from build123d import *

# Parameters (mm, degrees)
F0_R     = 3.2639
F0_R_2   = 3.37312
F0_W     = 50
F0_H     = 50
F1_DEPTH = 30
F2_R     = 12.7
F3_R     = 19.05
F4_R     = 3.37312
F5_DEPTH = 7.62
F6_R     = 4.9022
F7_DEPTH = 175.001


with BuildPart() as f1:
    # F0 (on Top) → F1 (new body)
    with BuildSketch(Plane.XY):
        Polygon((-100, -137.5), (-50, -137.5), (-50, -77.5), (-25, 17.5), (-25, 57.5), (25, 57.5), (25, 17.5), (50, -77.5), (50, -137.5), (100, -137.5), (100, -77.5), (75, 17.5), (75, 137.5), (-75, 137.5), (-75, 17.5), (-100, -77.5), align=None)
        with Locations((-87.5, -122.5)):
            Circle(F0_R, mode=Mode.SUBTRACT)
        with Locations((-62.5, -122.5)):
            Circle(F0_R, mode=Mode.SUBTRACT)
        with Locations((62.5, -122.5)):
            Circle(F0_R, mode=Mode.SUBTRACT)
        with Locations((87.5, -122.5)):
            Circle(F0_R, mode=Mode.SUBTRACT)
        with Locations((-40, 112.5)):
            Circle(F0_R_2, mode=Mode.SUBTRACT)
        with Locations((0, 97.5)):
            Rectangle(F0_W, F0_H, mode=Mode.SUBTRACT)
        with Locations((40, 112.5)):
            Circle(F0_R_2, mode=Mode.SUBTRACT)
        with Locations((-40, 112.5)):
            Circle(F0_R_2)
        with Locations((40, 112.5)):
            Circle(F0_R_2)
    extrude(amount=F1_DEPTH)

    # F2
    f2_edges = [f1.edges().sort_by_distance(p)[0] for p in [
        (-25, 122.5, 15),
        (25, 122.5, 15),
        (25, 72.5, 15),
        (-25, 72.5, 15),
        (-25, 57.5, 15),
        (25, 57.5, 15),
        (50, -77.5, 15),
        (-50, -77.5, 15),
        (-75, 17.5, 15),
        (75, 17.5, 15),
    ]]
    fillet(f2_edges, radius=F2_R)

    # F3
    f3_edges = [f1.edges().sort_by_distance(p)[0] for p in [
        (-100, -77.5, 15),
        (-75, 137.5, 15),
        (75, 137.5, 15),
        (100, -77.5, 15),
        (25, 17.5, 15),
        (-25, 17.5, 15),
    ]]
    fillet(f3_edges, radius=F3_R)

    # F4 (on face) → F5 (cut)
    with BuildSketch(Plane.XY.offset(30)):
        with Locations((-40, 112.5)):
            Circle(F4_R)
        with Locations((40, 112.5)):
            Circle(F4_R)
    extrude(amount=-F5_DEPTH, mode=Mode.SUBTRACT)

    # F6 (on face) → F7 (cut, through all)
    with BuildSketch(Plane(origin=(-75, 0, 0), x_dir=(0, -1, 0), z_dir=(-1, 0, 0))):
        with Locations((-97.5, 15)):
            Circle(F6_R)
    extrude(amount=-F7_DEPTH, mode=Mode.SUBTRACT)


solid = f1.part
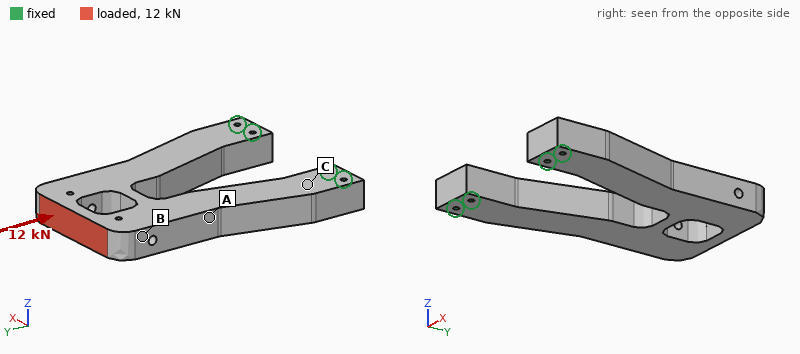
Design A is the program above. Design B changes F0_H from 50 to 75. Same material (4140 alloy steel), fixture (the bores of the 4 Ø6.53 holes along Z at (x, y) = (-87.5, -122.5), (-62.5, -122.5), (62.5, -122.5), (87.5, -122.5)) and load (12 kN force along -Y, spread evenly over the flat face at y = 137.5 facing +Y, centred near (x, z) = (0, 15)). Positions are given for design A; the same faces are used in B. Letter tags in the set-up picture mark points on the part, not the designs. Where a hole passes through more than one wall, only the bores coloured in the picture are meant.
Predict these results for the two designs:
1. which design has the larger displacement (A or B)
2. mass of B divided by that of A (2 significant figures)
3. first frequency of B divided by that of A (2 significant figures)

B
0.96
1.1
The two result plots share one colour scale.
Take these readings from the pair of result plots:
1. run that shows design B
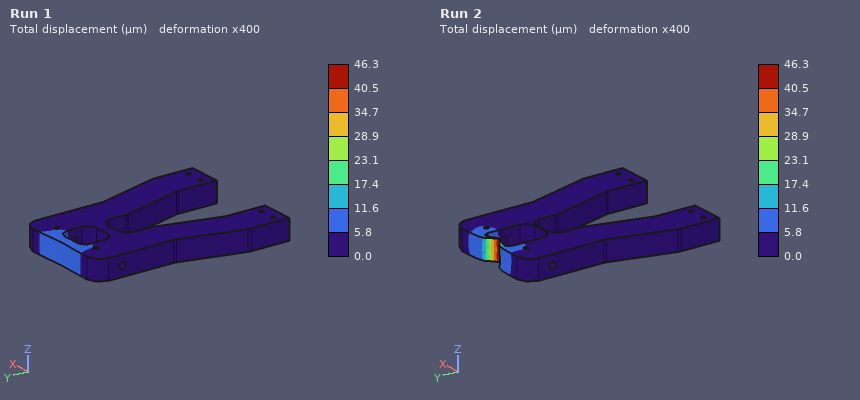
Run 2
